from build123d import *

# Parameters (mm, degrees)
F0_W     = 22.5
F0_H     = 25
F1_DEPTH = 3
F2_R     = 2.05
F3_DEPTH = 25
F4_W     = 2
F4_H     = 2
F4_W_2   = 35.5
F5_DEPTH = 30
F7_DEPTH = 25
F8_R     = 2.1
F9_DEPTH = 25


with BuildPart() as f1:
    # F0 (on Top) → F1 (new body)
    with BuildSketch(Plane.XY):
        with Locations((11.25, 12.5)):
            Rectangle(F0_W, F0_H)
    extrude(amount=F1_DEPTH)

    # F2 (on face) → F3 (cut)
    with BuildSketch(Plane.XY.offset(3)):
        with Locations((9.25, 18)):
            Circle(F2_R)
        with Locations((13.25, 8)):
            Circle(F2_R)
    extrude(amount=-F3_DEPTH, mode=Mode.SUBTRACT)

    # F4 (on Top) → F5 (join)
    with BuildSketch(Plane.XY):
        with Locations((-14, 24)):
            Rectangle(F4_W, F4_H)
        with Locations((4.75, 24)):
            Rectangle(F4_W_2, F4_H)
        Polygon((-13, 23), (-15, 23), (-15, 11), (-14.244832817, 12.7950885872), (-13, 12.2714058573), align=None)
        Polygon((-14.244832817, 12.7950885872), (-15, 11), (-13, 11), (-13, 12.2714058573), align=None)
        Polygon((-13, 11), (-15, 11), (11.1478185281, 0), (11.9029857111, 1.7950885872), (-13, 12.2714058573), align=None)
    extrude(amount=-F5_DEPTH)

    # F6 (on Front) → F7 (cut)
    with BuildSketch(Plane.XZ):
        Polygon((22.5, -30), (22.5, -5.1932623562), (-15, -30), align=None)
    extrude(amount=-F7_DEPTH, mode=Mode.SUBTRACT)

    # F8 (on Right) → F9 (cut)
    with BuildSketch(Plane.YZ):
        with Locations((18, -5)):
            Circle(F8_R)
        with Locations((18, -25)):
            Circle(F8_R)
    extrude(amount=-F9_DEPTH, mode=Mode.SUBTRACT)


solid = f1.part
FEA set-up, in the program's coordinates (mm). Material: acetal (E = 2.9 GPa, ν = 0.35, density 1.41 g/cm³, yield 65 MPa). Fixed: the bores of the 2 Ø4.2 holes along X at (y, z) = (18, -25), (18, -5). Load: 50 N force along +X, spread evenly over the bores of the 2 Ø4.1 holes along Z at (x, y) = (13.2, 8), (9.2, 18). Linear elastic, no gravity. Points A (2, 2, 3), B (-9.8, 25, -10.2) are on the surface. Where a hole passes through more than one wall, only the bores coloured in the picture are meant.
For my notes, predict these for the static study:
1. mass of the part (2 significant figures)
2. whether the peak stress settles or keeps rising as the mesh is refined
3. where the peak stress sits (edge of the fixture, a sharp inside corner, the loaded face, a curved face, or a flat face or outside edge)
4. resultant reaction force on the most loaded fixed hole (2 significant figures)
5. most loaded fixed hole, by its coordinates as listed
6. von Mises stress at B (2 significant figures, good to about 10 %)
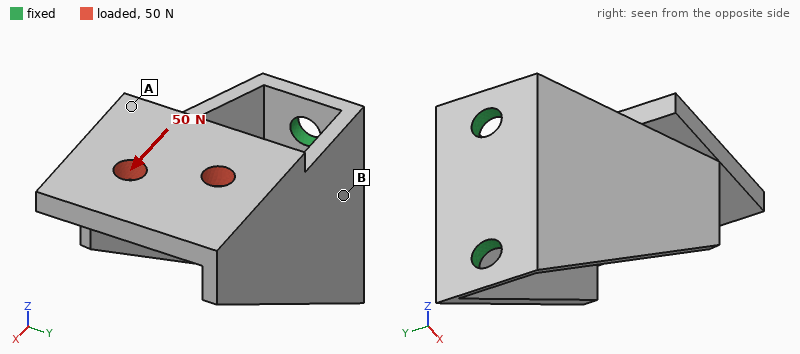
6.6 g
keeps rising
edge of the fixture
64 N
(18, -5)
4.1 MPa
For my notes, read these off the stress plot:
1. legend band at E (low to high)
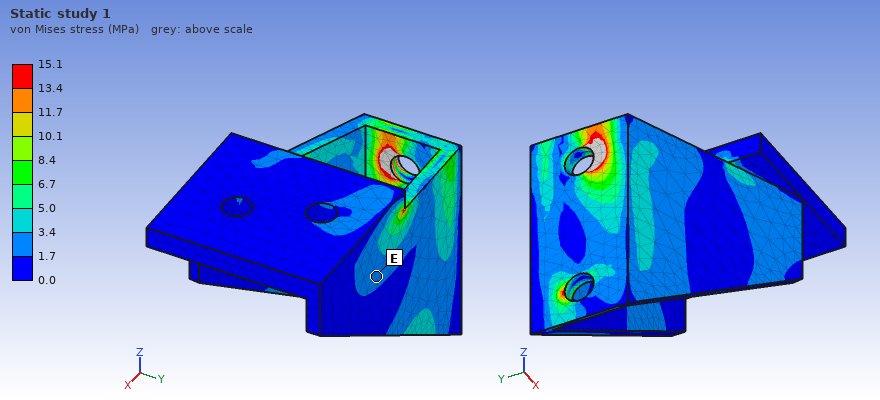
1.7 to 3.4 MPa
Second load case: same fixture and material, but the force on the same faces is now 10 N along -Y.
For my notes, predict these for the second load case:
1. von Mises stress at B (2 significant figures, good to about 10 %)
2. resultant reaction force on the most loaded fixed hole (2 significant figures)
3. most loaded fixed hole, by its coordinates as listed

3.3 MPa
12 N
(18, -5)
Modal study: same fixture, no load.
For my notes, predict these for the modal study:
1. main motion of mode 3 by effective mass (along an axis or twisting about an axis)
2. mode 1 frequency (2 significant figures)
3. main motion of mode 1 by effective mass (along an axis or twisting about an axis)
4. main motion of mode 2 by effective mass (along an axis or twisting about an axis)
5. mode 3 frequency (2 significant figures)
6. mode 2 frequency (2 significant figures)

along X
400 Hz
along Y
along Z
1800 Hz
1300 Hz
